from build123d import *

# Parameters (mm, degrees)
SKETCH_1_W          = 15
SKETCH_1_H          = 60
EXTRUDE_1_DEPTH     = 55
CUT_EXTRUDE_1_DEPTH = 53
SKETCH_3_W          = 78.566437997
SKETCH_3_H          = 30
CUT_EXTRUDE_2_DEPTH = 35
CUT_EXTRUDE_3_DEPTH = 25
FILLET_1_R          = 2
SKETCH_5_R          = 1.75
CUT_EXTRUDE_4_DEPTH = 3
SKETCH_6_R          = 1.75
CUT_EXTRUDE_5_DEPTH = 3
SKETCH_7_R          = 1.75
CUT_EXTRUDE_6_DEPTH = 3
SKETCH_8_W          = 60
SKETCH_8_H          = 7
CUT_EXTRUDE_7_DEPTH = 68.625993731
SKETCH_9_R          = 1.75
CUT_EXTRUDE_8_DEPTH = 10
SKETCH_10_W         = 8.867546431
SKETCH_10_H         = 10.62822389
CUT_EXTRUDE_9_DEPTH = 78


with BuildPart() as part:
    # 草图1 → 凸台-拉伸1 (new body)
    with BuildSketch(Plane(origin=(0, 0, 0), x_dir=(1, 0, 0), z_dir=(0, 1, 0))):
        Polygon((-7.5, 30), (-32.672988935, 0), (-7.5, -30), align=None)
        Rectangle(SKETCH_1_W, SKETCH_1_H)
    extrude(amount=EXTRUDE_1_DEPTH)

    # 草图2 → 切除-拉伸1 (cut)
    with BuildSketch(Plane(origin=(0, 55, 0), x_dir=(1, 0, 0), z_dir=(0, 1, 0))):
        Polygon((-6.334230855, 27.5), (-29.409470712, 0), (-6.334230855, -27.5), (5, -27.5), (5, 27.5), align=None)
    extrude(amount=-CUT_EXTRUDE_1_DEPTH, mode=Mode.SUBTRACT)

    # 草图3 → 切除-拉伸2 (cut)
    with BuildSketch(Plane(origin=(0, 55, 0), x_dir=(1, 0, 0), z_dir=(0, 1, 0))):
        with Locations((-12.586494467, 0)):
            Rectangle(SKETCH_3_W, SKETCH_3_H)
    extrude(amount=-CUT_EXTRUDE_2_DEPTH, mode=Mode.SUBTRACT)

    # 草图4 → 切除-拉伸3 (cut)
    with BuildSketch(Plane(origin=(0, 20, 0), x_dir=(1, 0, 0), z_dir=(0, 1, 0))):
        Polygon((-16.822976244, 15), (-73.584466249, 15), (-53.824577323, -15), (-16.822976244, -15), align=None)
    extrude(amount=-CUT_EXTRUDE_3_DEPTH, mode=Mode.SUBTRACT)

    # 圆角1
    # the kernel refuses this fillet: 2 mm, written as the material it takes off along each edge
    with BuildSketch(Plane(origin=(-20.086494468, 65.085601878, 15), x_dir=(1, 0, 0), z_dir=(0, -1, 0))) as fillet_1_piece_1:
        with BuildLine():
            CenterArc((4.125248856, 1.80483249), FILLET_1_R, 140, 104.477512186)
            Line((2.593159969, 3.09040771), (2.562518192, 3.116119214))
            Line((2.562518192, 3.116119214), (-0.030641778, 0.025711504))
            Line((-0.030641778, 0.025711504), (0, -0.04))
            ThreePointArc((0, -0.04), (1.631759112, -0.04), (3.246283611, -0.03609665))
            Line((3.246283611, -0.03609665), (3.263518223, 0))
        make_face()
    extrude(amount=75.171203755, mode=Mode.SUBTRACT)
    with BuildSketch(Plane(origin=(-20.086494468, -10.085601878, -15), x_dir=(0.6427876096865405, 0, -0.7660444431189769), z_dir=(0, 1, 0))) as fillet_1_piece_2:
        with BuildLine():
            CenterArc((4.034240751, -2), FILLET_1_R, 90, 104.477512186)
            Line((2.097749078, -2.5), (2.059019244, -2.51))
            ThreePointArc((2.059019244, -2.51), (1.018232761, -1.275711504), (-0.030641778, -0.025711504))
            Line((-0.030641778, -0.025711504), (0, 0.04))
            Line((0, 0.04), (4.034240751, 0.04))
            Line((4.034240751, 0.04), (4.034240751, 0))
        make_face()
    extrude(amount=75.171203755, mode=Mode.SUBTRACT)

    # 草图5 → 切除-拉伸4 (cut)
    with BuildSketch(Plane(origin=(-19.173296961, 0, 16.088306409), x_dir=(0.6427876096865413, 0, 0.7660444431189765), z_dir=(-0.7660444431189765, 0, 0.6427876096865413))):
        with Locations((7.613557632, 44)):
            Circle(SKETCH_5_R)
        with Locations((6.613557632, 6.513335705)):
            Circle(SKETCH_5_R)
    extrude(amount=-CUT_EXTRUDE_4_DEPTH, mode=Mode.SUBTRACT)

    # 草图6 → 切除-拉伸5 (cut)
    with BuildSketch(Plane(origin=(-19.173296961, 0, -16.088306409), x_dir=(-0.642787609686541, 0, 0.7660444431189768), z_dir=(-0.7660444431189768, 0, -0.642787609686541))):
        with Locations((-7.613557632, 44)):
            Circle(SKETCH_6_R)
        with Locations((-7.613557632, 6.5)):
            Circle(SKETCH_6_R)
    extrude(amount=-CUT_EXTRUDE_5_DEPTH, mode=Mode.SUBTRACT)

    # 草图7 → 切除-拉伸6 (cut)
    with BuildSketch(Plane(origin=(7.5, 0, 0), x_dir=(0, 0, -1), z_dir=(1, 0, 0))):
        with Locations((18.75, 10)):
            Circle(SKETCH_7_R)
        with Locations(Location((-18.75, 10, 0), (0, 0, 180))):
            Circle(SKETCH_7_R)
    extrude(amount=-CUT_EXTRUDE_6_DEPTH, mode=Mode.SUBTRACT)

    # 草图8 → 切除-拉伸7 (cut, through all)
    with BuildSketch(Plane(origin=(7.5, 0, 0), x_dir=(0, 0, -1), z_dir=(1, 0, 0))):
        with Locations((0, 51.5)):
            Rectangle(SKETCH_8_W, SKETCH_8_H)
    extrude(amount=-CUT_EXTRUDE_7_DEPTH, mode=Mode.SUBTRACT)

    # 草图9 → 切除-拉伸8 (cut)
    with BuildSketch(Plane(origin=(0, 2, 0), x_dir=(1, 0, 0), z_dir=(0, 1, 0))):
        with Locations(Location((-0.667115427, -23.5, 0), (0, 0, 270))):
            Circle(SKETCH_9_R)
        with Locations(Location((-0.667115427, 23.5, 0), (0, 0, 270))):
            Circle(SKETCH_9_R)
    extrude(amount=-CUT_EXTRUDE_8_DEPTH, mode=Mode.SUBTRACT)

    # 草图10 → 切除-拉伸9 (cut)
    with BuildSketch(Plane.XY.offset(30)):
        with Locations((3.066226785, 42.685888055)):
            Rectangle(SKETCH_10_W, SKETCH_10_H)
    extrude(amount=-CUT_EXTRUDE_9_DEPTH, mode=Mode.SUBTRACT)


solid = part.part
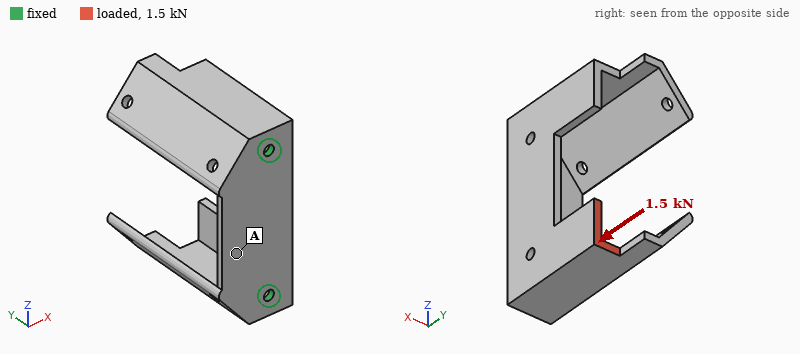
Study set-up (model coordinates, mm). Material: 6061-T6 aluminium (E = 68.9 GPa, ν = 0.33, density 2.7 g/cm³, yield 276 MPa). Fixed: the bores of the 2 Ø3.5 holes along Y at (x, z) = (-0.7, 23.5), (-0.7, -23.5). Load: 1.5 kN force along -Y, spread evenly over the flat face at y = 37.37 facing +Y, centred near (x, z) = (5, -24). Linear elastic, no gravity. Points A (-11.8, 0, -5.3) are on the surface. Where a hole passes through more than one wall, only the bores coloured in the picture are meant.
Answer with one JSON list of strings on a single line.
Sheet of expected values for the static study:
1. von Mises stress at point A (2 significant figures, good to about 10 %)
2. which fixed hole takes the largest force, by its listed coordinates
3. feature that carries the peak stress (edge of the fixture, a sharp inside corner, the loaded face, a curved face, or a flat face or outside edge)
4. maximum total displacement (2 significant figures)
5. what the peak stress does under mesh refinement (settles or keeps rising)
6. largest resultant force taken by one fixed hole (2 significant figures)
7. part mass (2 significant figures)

["30 MPa", "(-0.7, -23.5)", "edge of the fixture", "0.51 mm", "keeps rising", "1.5 kN", "34 g"]
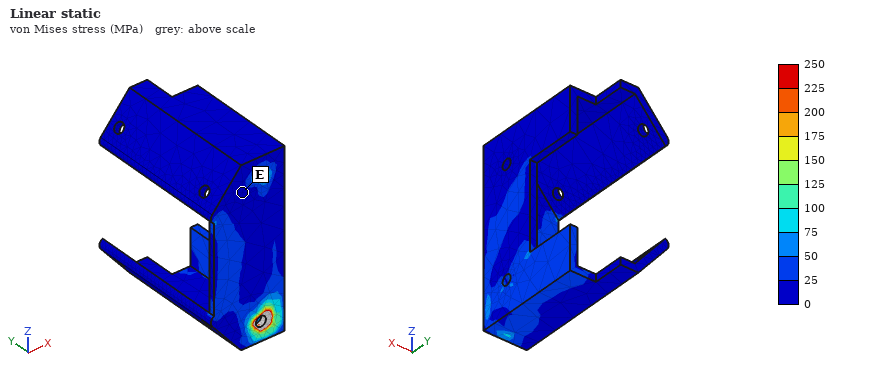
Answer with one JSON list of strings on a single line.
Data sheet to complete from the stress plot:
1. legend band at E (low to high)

["0 to 25 MPa"]
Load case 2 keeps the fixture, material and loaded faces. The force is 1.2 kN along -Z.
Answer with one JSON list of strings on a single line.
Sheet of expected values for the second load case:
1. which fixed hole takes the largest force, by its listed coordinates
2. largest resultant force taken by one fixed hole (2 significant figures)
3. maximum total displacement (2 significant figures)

["(-0.7, 23.5)", "1.5 kN", "0.48 mm"]
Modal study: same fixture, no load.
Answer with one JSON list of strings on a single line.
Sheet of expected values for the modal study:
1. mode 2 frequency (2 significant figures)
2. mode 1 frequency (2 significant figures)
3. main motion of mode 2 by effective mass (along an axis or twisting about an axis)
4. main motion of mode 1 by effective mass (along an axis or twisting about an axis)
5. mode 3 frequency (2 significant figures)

["1600 Hz", "1300 Hz", "twisting about Y", "along X", "2200 Hz"]
